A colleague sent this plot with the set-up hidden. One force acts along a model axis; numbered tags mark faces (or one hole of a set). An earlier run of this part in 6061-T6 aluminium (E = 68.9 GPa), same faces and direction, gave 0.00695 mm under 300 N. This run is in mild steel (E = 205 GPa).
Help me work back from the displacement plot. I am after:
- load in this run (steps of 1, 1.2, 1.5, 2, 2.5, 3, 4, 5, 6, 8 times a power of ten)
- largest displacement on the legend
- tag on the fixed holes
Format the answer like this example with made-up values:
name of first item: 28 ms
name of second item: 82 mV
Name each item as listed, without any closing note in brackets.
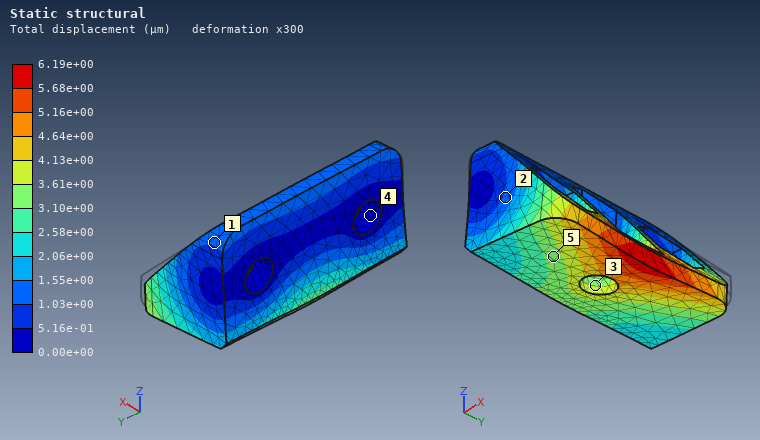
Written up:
load in this run: 800 N
largest displacement on the legend: 6.19e+00 µm
tag on the fixed holes: 4
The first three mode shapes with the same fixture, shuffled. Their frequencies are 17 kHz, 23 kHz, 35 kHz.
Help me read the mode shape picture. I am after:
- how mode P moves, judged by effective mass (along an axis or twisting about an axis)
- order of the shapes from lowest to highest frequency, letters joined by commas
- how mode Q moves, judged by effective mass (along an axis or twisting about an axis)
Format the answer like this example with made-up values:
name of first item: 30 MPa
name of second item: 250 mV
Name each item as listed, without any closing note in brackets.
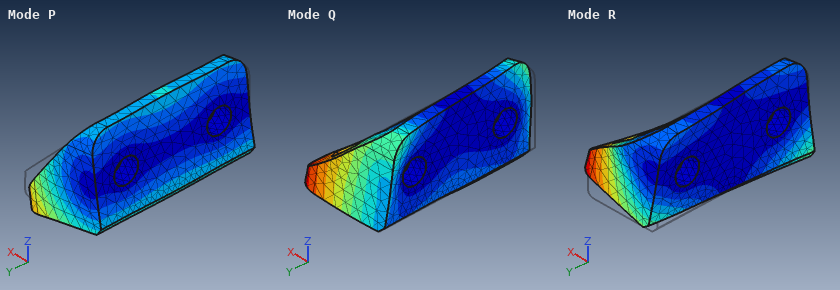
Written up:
how mode P moves, judged by effective mass: along Z
order of the shapes from lowest to highest frequency, letters joined by commas: P, R, Q
how mode Q moves, judged by effective mass: along Y
